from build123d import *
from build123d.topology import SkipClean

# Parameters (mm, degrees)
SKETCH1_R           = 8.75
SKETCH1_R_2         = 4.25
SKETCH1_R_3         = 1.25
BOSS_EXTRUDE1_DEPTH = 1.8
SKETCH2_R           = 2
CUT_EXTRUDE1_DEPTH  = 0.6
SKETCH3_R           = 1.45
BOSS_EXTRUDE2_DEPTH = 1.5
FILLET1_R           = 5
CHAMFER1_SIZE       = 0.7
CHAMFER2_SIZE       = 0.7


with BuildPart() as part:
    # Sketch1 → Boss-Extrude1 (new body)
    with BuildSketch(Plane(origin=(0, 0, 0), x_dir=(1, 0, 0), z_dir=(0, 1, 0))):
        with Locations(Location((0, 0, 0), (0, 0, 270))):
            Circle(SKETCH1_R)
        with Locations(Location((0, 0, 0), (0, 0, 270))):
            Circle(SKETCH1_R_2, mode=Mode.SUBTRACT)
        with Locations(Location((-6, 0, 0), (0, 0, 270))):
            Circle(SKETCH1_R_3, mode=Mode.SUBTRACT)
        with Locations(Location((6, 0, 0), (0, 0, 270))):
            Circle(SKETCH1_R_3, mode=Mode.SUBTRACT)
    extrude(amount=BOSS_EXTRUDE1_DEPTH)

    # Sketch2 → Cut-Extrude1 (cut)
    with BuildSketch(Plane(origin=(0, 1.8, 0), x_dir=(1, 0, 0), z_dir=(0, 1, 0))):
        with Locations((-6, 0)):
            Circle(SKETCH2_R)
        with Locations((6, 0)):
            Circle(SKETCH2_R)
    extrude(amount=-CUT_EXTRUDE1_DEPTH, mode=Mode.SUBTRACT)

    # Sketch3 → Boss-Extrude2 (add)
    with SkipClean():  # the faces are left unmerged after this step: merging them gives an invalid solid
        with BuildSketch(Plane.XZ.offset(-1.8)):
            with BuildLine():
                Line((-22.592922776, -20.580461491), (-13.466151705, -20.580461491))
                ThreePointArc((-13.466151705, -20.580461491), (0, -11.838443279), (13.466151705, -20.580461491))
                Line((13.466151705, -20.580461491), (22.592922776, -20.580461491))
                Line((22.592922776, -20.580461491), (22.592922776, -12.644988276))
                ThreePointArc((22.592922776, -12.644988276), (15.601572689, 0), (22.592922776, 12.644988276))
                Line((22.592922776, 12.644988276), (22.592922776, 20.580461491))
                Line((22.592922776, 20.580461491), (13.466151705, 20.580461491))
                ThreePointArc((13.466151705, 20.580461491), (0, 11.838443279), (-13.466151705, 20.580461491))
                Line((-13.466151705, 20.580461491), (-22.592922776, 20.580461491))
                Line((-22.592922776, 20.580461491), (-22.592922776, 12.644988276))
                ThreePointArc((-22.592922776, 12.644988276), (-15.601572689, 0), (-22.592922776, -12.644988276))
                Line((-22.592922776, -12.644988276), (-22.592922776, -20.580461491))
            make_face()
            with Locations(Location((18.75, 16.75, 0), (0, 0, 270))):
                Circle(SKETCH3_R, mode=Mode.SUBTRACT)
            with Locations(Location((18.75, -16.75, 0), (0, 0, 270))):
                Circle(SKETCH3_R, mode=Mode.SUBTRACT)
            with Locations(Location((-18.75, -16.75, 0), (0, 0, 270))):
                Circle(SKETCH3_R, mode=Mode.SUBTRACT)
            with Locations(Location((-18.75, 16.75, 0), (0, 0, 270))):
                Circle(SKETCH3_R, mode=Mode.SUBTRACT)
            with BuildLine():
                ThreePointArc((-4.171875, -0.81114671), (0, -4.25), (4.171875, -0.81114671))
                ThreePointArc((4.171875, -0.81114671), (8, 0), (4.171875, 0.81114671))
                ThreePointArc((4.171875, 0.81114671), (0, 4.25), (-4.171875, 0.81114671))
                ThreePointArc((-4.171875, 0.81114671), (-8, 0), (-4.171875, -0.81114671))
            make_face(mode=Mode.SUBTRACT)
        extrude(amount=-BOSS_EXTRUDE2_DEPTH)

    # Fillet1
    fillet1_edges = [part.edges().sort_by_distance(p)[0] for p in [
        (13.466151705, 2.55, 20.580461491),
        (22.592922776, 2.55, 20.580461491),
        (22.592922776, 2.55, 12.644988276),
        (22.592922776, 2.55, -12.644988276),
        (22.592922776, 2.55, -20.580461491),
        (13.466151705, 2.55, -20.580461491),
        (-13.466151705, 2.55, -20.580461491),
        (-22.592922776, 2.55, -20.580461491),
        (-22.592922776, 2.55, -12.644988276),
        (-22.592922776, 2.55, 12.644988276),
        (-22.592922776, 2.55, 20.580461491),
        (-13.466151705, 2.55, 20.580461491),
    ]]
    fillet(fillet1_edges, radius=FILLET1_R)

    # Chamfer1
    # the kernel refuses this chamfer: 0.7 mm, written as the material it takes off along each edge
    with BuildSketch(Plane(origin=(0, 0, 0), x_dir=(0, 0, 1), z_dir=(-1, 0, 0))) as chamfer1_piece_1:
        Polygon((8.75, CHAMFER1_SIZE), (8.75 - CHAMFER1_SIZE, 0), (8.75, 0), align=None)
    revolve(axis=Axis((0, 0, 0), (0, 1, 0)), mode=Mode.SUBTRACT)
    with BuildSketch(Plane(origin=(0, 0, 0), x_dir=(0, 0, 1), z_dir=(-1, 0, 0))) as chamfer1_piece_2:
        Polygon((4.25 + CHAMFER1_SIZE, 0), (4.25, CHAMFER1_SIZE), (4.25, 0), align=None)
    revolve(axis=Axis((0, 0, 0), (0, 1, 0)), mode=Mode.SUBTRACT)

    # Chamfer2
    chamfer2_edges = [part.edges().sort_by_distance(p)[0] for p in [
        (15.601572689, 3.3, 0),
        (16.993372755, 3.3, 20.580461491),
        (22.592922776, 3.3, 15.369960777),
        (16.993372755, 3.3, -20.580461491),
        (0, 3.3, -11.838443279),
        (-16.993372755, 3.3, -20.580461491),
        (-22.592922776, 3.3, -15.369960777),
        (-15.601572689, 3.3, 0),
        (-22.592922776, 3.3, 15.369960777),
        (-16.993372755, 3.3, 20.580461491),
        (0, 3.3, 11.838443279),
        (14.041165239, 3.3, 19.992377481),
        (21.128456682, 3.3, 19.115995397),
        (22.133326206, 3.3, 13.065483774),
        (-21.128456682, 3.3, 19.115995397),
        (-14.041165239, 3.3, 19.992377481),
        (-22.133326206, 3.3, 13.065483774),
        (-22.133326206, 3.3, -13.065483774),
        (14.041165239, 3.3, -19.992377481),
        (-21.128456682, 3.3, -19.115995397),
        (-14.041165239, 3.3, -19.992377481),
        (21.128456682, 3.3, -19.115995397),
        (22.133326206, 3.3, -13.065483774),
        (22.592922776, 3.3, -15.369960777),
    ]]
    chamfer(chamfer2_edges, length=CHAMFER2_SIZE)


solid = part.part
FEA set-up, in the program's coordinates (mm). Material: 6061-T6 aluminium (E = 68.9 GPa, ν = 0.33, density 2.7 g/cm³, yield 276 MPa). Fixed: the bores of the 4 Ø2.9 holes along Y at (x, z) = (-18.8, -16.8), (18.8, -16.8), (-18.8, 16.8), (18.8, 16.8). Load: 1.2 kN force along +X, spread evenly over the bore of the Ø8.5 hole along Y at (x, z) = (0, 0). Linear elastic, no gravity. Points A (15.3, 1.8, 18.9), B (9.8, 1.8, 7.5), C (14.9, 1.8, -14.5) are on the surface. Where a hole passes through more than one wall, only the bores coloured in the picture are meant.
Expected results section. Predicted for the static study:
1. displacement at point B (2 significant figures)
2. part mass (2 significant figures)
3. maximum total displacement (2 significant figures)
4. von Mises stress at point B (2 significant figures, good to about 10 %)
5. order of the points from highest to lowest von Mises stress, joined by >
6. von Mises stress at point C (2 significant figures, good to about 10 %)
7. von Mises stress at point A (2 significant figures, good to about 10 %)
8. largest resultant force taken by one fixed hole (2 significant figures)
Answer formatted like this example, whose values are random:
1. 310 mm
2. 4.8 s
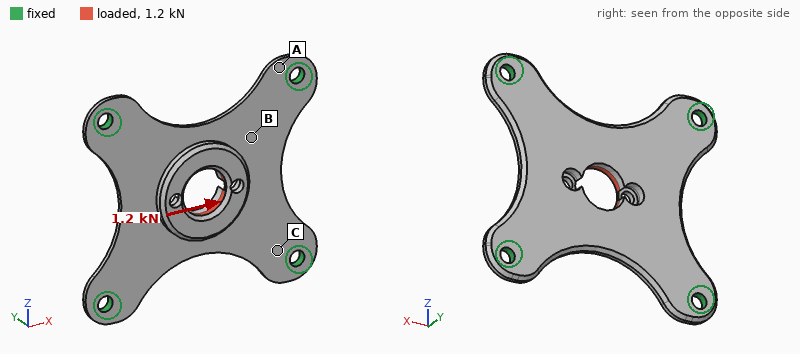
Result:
1. 24 µm
2. 5.2 g
3. 36 µm
4. 47 MPa
5. B > C > A
6. 34 MPa
7. 8.6 MPa
8. 370 N
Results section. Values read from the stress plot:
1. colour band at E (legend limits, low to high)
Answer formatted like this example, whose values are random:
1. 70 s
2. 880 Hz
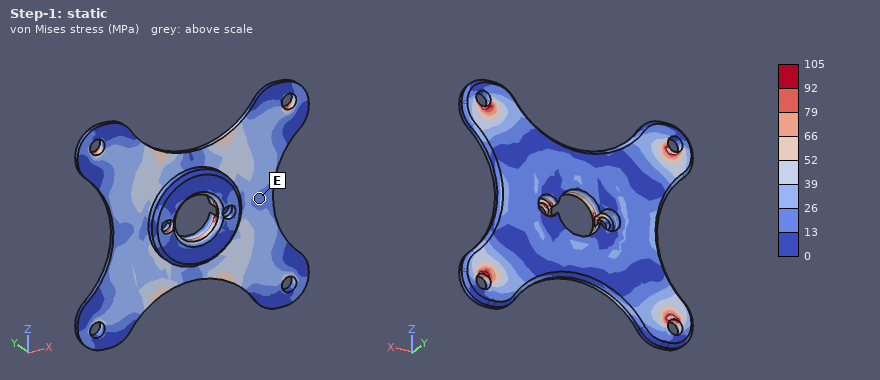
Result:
1. 13 to 26 MPa
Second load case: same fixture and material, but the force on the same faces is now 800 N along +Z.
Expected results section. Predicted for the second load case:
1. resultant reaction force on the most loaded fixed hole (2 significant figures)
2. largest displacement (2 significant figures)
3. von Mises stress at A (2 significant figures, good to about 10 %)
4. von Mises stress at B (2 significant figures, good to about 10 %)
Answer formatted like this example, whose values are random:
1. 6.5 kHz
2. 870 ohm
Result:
1. 260 N
2. 34 µm
3. 8.2 MPa
4. 33 MPa
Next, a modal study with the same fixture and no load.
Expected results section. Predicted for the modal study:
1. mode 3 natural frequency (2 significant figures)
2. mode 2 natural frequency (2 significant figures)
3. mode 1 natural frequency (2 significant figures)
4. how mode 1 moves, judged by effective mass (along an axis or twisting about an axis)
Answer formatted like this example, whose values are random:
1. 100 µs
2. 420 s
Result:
1. 8500 Hz
2. 8400 Hz
3. 4400 Hz
4. along Y
